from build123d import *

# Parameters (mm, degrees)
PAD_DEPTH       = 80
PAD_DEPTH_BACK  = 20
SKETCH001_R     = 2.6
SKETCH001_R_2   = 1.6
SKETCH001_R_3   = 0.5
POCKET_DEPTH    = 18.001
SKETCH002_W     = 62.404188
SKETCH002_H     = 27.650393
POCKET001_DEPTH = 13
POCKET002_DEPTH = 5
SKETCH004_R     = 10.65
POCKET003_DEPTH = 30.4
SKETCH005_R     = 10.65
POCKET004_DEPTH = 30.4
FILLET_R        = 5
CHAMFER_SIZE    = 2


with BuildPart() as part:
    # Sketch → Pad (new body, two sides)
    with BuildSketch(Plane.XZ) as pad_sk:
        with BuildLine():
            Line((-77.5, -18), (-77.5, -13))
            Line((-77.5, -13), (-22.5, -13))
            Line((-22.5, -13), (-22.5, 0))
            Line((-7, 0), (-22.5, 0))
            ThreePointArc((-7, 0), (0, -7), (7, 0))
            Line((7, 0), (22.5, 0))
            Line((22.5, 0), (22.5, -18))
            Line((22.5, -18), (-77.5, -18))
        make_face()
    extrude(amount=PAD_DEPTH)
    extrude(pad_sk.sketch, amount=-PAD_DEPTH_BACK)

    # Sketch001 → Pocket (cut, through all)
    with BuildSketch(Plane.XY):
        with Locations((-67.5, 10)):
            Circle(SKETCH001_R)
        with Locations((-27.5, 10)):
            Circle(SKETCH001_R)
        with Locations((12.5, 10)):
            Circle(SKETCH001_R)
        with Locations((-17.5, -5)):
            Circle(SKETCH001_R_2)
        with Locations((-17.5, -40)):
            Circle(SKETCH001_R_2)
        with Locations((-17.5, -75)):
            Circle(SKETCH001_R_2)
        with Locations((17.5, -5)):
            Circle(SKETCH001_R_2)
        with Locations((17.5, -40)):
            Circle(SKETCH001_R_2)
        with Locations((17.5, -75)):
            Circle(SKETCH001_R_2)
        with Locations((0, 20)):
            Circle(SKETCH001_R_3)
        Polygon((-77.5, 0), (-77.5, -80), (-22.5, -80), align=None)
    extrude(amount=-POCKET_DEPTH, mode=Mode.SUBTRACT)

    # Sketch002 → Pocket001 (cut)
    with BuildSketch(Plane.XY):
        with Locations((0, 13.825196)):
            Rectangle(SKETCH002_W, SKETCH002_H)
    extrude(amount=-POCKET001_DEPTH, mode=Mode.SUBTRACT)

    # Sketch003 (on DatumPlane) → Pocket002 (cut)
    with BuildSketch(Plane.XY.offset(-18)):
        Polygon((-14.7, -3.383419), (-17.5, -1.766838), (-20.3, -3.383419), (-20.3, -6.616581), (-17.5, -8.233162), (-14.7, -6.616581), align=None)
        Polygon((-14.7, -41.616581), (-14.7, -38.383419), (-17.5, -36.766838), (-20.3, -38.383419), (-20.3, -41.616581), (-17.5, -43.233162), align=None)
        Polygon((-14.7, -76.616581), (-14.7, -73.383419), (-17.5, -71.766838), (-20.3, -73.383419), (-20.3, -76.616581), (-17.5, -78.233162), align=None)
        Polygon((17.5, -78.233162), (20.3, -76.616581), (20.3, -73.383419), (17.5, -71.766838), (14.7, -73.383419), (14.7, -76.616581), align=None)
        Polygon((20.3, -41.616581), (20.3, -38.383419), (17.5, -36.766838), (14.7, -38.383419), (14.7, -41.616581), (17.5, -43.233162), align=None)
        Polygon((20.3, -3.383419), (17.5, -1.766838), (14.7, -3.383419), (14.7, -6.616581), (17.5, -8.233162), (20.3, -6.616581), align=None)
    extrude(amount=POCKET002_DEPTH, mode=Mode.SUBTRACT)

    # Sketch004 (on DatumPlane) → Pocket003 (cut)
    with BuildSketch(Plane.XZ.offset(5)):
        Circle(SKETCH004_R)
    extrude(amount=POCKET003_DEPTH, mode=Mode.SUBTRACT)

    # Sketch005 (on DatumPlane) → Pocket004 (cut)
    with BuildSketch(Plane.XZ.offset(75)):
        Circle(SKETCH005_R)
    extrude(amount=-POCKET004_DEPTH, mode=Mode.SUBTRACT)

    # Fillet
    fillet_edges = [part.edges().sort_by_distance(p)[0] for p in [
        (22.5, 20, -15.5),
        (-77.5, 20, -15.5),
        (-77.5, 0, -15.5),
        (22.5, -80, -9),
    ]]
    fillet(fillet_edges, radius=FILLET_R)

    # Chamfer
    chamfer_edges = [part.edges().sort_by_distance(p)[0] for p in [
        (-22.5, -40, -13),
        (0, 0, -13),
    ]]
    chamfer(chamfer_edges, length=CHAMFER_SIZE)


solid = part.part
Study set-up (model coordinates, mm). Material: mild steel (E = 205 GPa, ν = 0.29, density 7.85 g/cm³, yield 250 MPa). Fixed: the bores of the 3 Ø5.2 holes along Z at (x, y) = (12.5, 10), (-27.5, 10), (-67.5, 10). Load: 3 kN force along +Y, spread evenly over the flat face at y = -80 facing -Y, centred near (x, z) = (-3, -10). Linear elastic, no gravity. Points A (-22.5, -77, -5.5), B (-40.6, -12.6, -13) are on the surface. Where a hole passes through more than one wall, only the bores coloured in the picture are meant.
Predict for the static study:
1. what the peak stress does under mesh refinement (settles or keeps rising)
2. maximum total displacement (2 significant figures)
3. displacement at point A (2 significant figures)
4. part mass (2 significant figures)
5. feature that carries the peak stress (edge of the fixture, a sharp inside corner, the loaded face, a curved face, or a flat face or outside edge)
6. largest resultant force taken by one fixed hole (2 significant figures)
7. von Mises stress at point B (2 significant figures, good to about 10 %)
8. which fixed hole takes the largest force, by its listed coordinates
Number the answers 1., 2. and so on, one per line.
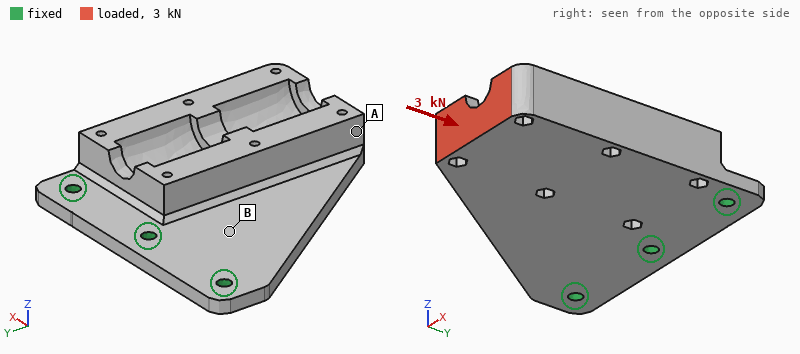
1. keeps rising
2. 0.13 mm
3. 0.11 mm
4. 560 g
5. edge of the fixture
6. 1.8 kN
7. 17 MPa
8. (12.5, 10)
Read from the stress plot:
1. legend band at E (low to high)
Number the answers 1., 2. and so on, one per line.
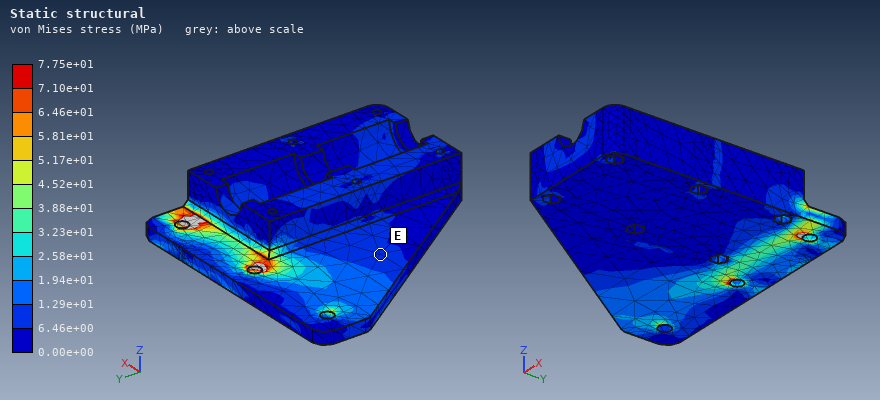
1. 6.46e+00 to 1.29e+01 MPa
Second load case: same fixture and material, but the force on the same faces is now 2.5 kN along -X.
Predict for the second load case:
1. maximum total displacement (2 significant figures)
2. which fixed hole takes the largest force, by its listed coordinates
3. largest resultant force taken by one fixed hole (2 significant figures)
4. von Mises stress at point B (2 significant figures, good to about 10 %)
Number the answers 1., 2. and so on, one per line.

1. 33 µm
2. (12.5, 10)
3. 3.4 kN
4. 16 MPa
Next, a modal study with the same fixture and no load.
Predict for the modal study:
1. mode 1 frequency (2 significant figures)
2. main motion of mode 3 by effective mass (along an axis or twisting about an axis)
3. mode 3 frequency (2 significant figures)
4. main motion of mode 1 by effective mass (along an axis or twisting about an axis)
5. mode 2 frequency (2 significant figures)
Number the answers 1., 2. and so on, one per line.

1. 510 Hz
2. along X
3. 4700 Hz
4. along Z
5. 2800 Hz
